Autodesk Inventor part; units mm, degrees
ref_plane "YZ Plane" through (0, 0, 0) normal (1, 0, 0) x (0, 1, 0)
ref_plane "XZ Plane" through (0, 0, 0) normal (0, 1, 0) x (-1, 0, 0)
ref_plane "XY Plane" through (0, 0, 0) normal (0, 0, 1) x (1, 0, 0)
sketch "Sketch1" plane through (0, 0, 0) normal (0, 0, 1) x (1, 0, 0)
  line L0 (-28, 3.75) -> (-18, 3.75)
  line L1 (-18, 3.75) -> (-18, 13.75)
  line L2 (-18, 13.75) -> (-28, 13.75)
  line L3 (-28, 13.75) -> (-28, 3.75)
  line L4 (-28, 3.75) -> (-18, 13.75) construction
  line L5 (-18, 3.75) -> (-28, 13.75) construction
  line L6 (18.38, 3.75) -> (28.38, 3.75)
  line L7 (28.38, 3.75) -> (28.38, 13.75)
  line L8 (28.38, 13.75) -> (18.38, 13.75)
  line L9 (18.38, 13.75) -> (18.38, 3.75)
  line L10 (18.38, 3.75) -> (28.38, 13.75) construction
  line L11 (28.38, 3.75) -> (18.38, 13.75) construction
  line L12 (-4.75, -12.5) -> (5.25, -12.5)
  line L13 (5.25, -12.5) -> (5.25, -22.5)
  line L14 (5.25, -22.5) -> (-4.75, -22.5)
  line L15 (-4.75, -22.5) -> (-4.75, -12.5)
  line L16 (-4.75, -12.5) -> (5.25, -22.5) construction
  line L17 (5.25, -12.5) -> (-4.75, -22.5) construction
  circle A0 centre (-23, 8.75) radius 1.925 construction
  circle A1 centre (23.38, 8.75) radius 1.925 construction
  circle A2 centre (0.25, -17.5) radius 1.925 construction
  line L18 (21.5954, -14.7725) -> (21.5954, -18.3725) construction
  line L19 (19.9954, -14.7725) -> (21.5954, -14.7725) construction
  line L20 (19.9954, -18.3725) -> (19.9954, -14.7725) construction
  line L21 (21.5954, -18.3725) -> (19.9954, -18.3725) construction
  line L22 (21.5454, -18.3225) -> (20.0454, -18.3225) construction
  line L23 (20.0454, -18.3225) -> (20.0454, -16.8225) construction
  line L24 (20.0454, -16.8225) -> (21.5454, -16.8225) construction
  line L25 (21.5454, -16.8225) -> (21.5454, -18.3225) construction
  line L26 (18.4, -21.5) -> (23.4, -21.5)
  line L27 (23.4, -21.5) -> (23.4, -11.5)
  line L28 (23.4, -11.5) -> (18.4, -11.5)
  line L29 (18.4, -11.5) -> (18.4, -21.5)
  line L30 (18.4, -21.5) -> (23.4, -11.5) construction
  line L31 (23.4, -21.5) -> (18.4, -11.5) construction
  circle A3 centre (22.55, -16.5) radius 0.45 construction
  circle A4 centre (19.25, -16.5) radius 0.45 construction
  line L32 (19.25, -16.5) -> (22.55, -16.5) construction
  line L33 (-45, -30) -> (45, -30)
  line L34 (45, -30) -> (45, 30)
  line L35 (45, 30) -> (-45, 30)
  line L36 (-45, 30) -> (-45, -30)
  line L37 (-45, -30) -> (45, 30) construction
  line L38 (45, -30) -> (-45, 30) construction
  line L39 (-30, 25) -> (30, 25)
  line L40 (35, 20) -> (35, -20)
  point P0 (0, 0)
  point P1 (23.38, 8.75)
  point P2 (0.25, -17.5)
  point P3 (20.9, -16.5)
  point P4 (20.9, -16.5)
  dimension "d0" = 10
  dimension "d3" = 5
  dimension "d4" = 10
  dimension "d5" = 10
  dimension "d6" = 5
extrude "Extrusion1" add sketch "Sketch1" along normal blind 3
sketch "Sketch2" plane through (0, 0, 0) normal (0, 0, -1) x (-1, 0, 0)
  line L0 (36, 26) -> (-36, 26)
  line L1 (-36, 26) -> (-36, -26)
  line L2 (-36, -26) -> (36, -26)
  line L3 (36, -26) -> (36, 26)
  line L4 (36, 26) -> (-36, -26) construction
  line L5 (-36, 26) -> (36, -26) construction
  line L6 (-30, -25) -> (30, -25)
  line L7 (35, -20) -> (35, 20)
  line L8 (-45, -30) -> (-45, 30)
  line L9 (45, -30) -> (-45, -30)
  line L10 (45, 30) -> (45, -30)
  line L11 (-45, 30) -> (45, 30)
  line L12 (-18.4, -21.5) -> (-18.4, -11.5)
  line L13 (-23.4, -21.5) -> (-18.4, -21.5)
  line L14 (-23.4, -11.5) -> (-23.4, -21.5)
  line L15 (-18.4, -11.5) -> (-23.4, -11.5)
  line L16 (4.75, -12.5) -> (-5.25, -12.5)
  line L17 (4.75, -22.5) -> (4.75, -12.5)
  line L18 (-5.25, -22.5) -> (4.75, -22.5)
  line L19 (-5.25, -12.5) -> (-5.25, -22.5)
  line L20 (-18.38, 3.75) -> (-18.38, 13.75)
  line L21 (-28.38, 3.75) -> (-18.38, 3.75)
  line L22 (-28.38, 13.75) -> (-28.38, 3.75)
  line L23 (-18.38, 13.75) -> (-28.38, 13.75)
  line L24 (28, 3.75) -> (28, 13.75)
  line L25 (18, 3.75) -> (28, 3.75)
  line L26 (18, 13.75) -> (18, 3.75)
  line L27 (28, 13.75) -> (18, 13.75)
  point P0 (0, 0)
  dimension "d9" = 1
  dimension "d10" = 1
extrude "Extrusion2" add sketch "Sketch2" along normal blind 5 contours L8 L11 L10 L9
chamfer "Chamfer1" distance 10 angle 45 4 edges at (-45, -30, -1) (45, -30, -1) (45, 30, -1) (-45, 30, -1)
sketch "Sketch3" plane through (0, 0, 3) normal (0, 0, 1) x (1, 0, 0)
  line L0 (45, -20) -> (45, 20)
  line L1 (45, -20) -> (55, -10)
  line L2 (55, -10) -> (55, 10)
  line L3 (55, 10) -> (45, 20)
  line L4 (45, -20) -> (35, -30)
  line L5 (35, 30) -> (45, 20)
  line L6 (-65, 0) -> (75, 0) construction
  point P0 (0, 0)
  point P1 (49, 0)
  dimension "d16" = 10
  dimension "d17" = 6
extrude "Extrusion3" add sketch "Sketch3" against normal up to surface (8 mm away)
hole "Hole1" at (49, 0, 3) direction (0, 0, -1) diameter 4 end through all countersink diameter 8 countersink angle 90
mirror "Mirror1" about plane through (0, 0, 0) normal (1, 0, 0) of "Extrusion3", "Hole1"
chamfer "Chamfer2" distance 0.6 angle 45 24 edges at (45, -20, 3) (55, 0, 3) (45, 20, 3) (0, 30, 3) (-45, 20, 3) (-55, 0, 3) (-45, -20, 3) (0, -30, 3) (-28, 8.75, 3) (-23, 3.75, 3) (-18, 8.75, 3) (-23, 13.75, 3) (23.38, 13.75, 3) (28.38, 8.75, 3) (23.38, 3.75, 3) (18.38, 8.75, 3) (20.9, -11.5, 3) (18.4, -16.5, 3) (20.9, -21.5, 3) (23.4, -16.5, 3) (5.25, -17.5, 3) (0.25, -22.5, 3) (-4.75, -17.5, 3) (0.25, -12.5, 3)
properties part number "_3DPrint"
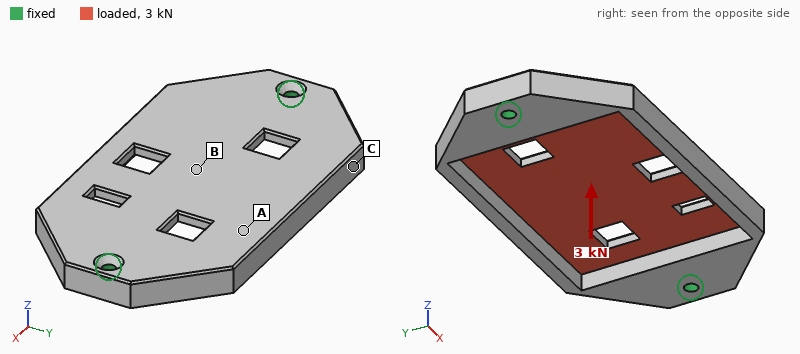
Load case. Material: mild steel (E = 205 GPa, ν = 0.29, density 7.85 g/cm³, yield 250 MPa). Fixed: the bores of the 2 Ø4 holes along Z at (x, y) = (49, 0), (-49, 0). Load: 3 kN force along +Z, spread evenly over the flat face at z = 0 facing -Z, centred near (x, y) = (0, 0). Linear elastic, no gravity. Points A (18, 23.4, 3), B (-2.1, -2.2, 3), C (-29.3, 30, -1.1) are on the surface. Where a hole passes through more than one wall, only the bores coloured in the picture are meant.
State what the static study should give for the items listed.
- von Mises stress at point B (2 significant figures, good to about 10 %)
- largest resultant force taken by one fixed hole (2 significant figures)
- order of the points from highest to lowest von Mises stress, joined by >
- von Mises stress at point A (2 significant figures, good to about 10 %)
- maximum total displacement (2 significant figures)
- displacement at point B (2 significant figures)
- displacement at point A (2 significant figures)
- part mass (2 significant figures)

94 MPa
2.1 kN
B > A > C
57 MPa
0.13 mm
0.12 mm
0.076 mm
210 g
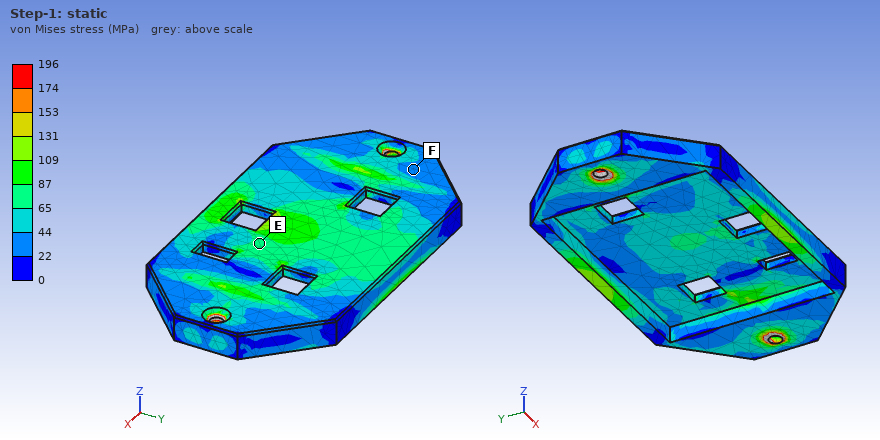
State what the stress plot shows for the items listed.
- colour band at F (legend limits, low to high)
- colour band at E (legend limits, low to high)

22 to 44 MPa
65 to 87 MPa
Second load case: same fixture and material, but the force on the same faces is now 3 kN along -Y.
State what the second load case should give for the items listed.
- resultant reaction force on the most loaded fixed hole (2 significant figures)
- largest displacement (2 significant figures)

1.5 kN
9.4 µm
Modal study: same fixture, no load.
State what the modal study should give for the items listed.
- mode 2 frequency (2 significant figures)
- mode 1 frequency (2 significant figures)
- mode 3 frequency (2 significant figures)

2800 Hz
2700 Hz
5600 Hz
